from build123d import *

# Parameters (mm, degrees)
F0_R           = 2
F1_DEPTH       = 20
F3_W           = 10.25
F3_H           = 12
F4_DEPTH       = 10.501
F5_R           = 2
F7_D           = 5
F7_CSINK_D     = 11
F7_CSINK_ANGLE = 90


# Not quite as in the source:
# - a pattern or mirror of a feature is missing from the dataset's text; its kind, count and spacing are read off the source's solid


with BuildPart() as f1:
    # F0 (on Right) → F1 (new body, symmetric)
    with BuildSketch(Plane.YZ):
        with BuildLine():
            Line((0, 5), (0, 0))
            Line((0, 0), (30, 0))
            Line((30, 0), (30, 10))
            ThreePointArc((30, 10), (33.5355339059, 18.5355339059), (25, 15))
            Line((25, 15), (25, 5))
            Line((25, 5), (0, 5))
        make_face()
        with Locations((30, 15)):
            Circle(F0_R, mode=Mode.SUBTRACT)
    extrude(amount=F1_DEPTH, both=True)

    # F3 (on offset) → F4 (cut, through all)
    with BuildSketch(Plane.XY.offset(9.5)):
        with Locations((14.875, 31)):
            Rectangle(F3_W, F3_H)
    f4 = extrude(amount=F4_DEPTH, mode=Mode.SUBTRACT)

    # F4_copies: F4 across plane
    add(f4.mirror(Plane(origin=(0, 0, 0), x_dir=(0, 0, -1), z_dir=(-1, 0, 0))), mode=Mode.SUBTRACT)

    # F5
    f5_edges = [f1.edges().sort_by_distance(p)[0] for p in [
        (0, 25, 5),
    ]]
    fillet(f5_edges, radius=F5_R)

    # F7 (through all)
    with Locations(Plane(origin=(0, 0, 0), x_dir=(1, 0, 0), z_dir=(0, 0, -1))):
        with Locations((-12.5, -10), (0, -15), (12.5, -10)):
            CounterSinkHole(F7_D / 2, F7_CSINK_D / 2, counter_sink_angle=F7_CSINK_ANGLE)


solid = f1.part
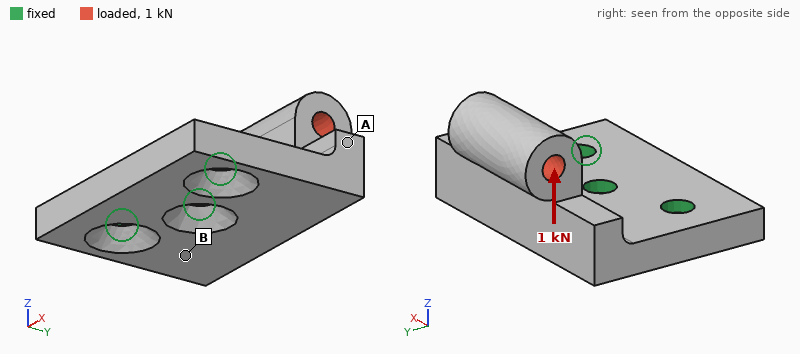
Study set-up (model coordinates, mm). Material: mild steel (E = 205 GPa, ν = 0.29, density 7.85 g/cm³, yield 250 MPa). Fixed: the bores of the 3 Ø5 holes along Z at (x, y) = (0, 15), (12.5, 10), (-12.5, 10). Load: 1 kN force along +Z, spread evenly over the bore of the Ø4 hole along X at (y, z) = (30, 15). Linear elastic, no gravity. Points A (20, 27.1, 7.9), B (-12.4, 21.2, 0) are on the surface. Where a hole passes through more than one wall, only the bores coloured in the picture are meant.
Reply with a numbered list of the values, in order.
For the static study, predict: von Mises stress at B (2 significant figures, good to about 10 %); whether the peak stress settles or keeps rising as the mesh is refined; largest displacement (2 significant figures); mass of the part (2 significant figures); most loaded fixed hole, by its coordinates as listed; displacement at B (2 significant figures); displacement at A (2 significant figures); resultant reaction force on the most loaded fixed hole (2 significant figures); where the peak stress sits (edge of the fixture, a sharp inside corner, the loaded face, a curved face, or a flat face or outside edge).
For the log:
1. 49 MPa
2. keeps rising
3. 61 µm
4. 61 g
5. (0, 15)
6. 14 µm
7. 27 µm
8. 1.5 kN
9. edge of the fixture
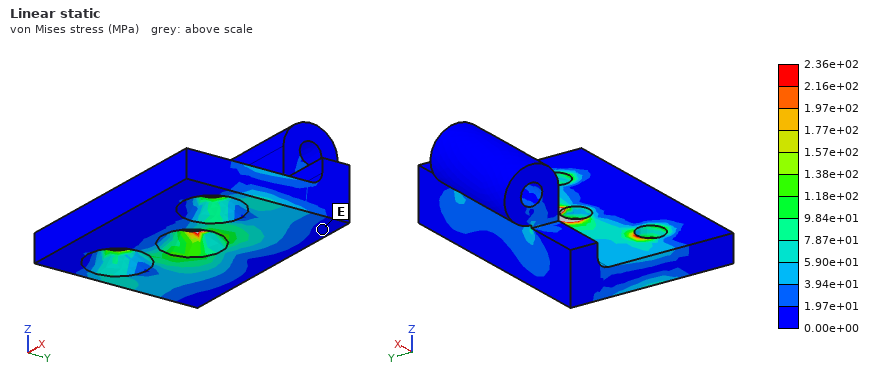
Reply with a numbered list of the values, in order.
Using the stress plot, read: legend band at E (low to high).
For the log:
1. 0.00e+00 to 1.97e+01 MPa
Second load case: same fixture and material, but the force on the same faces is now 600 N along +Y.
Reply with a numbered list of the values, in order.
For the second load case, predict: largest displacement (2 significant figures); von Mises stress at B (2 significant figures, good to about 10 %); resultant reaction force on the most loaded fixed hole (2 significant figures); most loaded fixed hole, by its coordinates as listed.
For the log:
1. 41 µm
2. 37 MPa
3. 660 N
4. (0, 15)
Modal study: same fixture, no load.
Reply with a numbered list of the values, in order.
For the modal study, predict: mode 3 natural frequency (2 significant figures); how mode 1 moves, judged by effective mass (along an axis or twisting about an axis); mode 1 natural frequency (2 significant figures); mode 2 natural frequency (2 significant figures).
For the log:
1. 14 kHz
2. along Z
3. 4700 Hz
4. 8100 Hz
